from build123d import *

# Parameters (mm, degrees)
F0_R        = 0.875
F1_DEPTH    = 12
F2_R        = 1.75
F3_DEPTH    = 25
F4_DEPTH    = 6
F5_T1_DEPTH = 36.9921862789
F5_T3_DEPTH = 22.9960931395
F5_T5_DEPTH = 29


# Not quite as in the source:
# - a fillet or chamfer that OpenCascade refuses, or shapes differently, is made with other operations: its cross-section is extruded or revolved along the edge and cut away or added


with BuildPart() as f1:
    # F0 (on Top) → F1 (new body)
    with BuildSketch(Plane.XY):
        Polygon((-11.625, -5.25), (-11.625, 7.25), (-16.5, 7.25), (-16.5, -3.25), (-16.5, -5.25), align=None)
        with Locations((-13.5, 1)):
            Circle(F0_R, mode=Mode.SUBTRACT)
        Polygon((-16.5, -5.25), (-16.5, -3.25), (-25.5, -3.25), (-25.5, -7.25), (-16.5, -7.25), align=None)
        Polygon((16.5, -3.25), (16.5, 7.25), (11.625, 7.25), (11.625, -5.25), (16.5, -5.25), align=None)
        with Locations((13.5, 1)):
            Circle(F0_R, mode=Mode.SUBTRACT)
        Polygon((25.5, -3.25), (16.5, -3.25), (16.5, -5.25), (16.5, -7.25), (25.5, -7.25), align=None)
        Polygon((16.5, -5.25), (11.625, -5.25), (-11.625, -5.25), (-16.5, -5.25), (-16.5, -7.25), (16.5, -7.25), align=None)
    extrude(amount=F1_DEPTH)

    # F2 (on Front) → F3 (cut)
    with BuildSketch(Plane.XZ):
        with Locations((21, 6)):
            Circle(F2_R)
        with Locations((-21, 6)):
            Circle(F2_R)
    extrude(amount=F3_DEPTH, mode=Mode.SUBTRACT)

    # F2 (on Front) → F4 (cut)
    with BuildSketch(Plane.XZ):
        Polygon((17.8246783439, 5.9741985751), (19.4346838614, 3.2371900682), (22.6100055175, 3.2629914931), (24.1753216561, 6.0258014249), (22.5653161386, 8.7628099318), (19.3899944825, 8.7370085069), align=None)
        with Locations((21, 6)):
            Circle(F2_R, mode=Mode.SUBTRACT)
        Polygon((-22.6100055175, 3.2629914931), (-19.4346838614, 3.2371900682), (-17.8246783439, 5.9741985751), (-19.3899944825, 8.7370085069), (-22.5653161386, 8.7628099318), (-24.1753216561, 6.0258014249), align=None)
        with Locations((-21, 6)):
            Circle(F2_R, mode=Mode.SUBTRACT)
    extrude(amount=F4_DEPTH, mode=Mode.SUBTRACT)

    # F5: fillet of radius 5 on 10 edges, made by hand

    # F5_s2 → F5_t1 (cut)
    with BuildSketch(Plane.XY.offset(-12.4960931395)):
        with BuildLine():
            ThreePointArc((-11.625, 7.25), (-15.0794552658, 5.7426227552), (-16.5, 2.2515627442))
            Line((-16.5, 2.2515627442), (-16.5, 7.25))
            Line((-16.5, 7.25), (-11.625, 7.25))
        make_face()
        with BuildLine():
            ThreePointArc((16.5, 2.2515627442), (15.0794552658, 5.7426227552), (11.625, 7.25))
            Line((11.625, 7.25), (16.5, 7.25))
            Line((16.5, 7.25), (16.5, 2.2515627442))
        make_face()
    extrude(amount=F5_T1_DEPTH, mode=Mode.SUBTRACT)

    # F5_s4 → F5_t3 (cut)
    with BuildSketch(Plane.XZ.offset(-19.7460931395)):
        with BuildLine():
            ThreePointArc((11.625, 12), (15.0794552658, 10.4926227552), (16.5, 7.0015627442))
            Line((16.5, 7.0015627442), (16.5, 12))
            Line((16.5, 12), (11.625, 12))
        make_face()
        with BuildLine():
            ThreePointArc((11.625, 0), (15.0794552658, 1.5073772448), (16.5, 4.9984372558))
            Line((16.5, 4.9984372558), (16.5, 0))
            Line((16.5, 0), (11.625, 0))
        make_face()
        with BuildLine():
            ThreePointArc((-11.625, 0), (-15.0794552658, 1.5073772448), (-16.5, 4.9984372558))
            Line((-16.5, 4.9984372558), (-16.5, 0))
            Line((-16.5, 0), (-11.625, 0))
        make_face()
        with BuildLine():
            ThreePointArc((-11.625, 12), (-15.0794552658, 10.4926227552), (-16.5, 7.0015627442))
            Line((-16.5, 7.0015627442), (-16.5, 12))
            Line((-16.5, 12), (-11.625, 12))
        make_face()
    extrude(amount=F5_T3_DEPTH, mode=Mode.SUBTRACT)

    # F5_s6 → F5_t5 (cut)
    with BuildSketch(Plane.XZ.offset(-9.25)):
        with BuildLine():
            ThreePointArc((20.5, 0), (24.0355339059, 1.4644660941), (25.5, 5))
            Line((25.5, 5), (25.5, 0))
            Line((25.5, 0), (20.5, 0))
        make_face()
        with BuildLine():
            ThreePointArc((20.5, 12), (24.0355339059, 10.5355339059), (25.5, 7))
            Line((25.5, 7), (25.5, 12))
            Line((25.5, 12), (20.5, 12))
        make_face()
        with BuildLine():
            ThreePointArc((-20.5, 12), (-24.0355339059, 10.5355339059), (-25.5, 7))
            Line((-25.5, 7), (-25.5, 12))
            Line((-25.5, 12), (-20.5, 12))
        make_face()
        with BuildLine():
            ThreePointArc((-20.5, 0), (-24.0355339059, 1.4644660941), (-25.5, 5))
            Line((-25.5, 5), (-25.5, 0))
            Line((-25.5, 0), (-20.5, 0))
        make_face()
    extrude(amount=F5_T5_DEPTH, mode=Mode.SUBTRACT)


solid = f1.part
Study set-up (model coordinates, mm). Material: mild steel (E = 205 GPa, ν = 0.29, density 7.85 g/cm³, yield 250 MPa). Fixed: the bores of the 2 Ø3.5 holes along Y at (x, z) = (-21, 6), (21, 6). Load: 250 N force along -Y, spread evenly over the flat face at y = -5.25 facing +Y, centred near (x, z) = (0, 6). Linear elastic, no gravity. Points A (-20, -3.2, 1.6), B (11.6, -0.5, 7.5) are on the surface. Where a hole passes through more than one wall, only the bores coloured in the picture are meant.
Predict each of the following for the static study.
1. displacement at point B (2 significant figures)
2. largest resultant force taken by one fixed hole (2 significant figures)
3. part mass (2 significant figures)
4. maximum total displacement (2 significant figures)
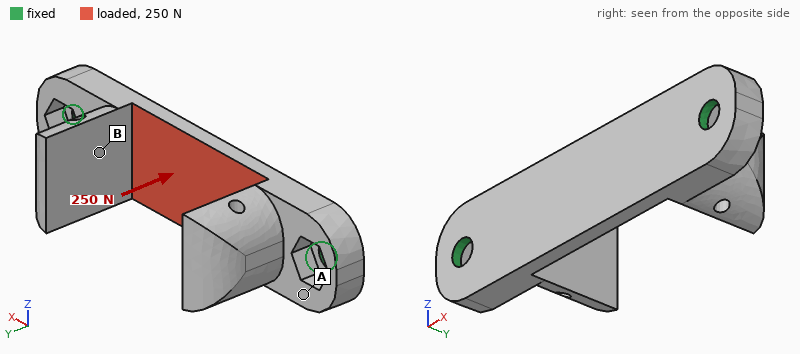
15 µm
130 N
20 g
28 µm
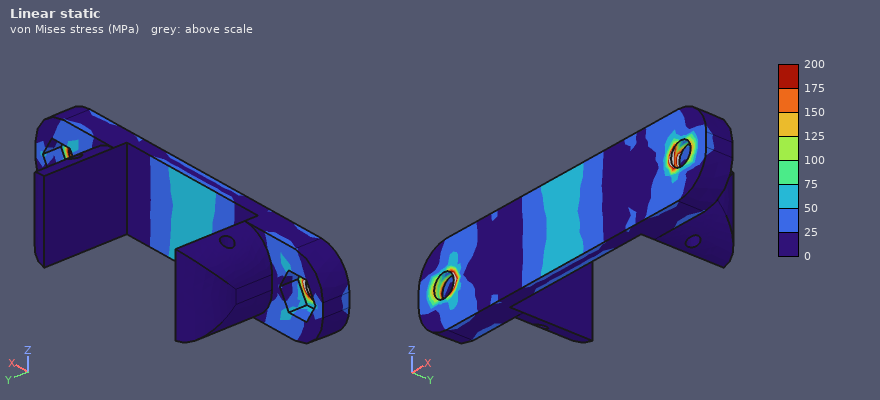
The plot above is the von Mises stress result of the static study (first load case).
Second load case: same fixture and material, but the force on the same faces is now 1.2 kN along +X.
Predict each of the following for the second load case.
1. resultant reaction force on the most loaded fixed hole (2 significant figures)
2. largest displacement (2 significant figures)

600 N
2.4 µm
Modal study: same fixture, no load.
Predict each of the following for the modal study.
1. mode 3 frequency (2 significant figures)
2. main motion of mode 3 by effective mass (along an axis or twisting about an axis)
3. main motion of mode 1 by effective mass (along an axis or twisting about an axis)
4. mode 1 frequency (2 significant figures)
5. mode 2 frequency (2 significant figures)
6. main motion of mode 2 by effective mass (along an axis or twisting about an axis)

8700 Hz
along X
along Y
5500 Hz
8200 Hz
along Z
